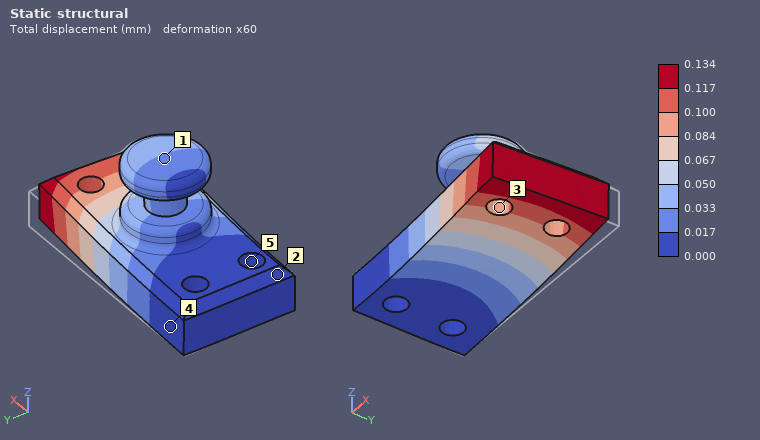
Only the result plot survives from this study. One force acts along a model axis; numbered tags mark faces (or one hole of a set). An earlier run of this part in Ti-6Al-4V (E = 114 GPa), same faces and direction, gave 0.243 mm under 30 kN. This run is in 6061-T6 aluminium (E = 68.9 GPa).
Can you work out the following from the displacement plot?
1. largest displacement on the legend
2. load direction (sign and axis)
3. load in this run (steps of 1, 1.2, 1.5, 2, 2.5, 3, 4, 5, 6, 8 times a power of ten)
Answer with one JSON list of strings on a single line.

["0.134 mm", "-Y", "10 kN"]
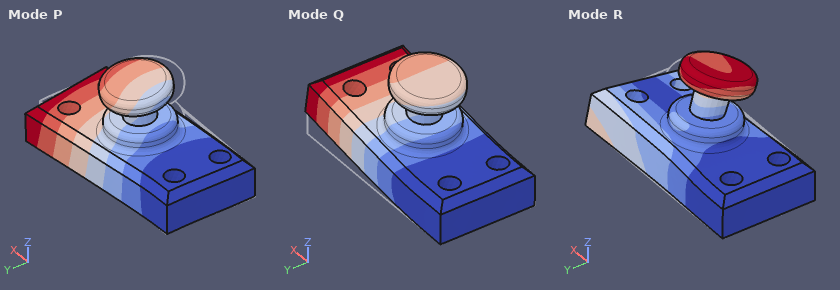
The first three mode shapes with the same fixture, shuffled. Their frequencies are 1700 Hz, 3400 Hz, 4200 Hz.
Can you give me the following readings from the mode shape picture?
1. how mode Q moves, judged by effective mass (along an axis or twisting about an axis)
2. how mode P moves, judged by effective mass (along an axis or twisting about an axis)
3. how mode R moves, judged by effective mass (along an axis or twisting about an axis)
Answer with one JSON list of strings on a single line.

["along Z", "along Y", "twisting about X"]
